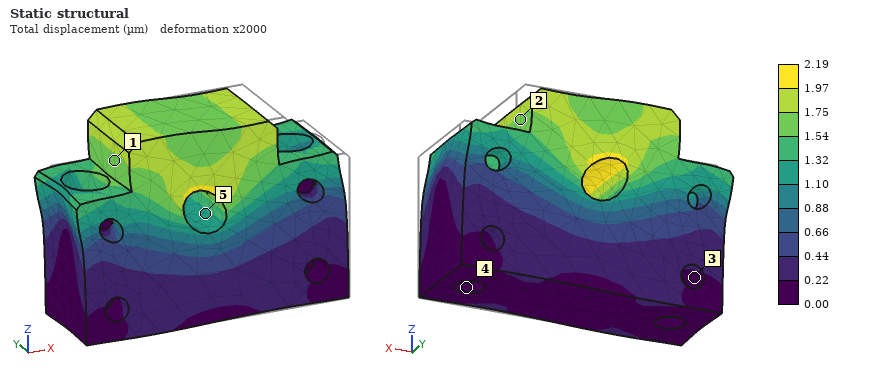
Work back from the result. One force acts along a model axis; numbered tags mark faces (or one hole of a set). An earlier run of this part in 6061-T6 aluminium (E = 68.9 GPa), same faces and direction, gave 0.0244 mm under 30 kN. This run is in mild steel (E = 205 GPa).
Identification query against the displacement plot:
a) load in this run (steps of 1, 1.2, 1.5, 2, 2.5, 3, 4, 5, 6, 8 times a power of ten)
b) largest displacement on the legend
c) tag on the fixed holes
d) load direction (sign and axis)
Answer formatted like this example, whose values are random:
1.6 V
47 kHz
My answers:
8 kN
2.19 µm
4
-X
